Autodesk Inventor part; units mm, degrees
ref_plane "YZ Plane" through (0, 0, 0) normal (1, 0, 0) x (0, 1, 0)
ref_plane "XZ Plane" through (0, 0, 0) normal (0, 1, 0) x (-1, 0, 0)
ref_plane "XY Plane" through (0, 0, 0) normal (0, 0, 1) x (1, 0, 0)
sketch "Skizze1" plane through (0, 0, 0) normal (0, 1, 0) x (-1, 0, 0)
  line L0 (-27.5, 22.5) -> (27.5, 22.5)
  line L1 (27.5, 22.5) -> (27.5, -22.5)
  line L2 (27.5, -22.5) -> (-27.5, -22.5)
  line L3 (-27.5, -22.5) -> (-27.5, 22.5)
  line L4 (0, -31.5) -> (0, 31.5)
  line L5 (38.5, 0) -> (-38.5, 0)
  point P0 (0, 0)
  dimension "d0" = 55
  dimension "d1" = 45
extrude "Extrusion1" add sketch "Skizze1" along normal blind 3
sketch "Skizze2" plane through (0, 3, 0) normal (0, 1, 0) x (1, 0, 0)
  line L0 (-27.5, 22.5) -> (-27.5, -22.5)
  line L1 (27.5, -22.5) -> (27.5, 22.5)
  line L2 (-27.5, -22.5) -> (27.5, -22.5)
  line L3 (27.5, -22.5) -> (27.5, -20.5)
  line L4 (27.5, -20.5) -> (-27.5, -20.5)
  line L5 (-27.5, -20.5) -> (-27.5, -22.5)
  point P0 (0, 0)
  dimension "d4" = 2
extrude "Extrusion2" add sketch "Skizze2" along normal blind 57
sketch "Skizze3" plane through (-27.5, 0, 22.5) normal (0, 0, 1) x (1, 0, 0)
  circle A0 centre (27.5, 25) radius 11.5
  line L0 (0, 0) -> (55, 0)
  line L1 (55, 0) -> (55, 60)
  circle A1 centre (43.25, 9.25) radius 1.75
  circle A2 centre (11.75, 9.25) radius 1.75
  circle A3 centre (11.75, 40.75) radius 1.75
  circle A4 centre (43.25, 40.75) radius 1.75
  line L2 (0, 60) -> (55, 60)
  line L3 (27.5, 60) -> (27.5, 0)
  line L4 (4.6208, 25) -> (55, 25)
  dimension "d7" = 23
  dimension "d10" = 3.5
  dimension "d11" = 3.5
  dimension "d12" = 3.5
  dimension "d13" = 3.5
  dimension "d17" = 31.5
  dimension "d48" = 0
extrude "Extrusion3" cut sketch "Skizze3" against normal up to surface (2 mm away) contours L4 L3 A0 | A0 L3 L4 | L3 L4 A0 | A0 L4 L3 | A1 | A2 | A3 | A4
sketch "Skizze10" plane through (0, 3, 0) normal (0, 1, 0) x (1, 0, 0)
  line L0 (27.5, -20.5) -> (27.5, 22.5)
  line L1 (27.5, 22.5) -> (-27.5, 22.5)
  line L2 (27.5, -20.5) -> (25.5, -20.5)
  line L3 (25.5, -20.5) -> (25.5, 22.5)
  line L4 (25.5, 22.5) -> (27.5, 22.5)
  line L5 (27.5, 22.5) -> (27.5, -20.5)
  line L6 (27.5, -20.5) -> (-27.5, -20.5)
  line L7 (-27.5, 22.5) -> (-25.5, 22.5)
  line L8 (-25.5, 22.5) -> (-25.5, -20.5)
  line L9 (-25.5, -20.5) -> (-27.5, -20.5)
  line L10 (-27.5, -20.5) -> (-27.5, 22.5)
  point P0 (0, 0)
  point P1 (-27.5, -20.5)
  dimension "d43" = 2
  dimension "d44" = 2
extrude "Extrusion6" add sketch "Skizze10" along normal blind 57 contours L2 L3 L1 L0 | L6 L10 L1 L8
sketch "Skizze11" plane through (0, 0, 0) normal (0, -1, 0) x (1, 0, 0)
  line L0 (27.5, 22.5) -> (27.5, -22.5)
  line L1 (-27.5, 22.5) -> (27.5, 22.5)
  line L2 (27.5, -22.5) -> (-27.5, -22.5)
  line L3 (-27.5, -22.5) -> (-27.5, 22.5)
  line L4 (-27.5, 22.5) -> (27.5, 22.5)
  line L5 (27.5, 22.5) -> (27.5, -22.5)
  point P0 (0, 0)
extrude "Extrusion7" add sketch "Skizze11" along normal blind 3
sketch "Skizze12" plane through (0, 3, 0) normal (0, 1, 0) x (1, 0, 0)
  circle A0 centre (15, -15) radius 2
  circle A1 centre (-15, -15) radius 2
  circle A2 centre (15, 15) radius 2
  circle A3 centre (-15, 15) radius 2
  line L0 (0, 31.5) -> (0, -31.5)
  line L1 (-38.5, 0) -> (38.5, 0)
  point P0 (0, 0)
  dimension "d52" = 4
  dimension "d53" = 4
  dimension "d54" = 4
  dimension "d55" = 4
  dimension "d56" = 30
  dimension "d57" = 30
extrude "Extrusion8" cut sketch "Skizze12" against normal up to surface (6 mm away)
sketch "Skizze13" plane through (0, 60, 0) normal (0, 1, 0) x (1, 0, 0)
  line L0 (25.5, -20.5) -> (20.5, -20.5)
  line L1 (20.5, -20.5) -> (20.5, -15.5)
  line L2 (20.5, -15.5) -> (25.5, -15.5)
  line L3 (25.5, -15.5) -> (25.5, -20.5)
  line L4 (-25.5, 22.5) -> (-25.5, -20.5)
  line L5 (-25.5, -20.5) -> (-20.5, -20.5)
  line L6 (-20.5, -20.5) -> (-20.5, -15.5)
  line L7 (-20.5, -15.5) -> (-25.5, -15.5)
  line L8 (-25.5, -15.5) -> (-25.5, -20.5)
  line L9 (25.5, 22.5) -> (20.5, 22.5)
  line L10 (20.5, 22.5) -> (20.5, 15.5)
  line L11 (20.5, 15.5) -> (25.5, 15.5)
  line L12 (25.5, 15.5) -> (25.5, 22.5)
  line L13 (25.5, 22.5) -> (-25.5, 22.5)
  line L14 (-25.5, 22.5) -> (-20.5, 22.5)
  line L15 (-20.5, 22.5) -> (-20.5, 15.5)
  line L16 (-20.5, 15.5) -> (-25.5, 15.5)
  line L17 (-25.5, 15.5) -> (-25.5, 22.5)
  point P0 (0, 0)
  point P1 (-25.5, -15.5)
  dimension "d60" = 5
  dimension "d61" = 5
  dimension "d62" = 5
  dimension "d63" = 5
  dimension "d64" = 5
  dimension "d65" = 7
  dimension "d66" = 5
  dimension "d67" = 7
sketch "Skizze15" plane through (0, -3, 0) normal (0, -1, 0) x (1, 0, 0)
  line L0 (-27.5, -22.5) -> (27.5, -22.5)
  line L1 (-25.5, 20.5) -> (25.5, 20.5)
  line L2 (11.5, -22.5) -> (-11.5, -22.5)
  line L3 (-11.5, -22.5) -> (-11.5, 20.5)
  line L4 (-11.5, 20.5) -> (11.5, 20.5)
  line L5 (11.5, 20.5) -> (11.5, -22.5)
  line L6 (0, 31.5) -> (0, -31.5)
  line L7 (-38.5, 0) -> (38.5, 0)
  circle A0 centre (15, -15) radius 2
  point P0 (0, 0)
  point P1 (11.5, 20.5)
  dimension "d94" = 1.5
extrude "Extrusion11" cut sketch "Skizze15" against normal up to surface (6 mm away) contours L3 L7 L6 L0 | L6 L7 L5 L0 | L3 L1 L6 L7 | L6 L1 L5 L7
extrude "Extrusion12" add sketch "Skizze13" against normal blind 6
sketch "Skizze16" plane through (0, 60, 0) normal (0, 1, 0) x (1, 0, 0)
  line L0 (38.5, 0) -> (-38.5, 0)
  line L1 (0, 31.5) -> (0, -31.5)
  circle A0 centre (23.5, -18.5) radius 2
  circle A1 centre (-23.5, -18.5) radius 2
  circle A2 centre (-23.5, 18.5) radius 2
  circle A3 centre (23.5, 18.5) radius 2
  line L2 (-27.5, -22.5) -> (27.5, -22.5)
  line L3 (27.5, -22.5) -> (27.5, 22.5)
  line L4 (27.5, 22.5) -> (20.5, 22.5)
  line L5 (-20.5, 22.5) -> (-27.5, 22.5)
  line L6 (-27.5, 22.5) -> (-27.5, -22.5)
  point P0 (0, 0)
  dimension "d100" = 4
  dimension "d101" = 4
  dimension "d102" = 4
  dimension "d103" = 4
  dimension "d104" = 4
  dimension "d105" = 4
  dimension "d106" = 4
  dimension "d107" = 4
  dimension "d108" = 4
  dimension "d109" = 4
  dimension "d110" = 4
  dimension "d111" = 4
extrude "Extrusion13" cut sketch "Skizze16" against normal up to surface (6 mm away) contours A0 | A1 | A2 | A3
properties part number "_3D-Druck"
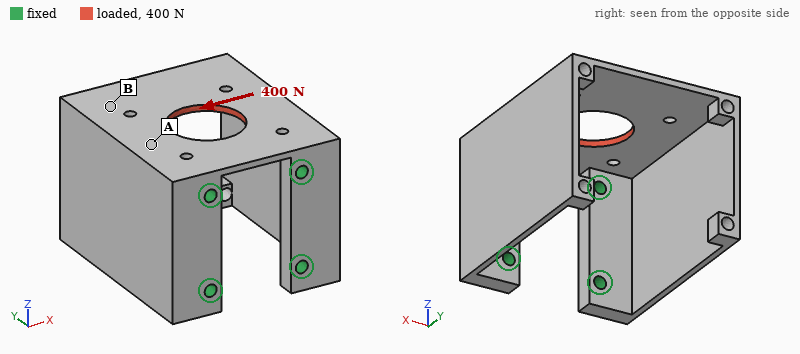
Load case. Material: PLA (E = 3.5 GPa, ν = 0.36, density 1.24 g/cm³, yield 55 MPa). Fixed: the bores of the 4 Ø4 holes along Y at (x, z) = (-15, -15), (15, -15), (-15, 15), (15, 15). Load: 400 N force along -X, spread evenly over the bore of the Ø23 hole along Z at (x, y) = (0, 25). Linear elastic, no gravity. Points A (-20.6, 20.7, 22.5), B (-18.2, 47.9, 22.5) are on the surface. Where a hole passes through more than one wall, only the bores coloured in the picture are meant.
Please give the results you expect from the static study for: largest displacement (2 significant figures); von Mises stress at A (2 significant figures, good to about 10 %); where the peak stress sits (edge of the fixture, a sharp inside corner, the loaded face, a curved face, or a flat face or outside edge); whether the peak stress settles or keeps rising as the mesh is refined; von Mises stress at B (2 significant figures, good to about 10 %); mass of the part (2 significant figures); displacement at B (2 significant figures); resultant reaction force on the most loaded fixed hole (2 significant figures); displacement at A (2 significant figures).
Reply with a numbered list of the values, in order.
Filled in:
1. 0.47 mm
2. 6.9 MPa
3. edge of the fixture
4. keeps rising
5. 2.3 MPa
6. 30 g
7. 0.37 mm
8. 340 N
9. 0.21 mm
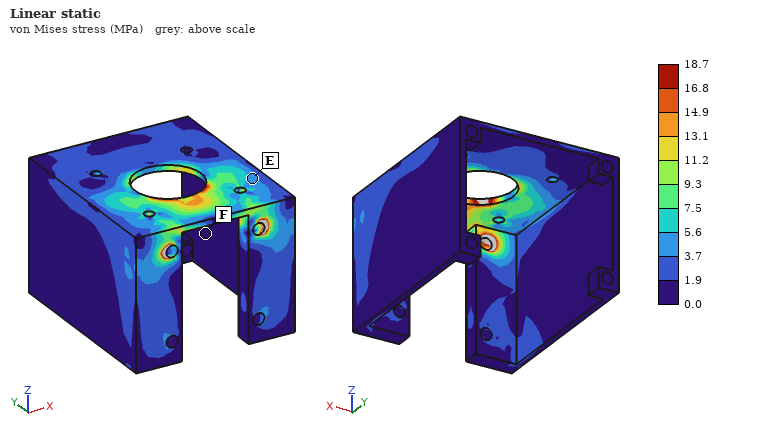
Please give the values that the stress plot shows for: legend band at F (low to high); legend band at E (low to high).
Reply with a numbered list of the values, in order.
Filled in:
1. 0.0 to 1.9 MPa
2. 3.7 to 5.6 MPa
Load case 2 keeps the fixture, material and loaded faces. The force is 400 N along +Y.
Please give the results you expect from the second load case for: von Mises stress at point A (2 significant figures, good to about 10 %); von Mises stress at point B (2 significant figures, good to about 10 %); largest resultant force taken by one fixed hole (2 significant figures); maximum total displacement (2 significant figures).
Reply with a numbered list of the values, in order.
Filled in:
1. 2.7 MPa
2. 1.9 MPa
3. 210 N
4. 0.13 mm
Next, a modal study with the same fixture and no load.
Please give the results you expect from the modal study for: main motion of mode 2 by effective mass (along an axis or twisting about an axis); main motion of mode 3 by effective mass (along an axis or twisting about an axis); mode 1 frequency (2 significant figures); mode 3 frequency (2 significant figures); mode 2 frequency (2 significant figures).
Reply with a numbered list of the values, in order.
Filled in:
1. along X
2. along Z
3. 320 Hz
4. 940 Hz
5. 360 Hz
